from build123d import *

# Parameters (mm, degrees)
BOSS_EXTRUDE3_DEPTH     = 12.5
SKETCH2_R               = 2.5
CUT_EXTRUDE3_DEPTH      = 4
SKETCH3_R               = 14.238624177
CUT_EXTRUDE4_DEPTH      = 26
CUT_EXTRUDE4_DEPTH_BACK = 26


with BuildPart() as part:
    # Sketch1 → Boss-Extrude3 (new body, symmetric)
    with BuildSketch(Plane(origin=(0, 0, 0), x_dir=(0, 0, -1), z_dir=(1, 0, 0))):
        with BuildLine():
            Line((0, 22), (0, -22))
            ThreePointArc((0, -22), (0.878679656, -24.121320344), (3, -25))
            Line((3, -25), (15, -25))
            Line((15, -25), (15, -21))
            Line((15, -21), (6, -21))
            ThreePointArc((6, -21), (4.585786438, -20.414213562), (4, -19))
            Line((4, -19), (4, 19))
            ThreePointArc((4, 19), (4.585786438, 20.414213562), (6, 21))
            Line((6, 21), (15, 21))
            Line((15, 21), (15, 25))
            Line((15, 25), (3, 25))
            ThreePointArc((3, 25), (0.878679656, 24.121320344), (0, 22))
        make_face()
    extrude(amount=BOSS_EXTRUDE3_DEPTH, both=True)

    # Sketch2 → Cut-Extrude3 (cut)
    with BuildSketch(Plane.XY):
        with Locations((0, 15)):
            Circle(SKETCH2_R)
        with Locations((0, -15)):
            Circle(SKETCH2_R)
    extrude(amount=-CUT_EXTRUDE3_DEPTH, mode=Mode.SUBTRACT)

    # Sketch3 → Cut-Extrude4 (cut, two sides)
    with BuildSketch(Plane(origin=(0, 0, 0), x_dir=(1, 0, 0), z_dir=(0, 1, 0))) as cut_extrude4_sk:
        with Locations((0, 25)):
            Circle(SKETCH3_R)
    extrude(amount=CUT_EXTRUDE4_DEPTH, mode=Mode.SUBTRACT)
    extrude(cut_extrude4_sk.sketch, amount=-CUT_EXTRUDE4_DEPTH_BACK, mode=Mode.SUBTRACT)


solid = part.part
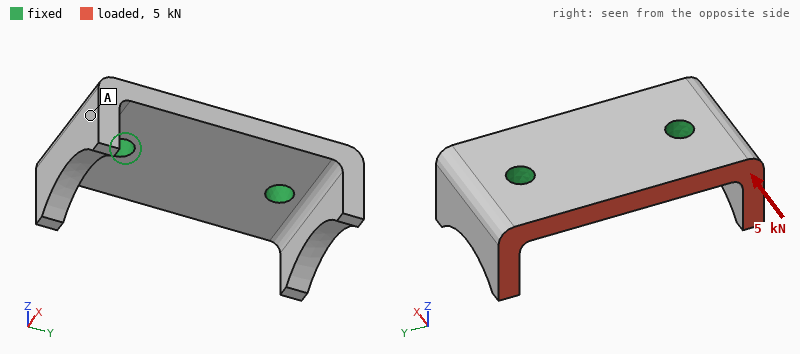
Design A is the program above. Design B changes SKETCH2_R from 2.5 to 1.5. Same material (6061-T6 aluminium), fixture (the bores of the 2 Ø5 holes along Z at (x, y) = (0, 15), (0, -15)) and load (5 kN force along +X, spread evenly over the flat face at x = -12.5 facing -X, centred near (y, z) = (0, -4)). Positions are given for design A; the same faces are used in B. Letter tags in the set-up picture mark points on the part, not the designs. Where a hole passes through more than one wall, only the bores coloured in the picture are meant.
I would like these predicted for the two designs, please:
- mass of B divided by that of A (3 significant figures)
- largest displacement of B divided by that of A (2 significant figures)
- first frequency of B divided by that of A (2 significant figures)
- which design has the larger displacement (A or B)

1.02
1.4
0.78
B
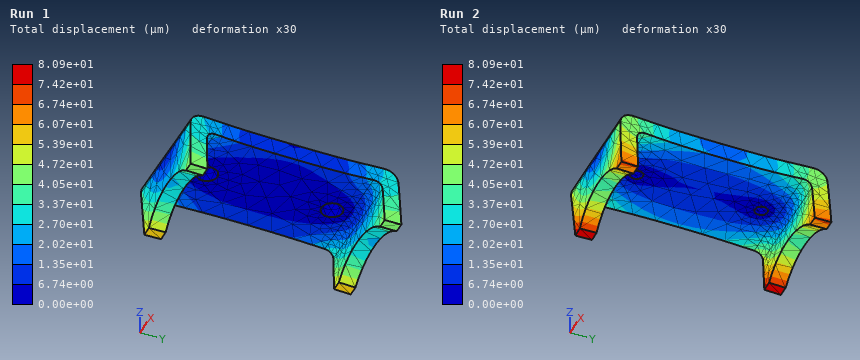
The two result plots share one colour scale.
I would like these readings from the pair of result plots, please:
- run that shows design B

Run 2
